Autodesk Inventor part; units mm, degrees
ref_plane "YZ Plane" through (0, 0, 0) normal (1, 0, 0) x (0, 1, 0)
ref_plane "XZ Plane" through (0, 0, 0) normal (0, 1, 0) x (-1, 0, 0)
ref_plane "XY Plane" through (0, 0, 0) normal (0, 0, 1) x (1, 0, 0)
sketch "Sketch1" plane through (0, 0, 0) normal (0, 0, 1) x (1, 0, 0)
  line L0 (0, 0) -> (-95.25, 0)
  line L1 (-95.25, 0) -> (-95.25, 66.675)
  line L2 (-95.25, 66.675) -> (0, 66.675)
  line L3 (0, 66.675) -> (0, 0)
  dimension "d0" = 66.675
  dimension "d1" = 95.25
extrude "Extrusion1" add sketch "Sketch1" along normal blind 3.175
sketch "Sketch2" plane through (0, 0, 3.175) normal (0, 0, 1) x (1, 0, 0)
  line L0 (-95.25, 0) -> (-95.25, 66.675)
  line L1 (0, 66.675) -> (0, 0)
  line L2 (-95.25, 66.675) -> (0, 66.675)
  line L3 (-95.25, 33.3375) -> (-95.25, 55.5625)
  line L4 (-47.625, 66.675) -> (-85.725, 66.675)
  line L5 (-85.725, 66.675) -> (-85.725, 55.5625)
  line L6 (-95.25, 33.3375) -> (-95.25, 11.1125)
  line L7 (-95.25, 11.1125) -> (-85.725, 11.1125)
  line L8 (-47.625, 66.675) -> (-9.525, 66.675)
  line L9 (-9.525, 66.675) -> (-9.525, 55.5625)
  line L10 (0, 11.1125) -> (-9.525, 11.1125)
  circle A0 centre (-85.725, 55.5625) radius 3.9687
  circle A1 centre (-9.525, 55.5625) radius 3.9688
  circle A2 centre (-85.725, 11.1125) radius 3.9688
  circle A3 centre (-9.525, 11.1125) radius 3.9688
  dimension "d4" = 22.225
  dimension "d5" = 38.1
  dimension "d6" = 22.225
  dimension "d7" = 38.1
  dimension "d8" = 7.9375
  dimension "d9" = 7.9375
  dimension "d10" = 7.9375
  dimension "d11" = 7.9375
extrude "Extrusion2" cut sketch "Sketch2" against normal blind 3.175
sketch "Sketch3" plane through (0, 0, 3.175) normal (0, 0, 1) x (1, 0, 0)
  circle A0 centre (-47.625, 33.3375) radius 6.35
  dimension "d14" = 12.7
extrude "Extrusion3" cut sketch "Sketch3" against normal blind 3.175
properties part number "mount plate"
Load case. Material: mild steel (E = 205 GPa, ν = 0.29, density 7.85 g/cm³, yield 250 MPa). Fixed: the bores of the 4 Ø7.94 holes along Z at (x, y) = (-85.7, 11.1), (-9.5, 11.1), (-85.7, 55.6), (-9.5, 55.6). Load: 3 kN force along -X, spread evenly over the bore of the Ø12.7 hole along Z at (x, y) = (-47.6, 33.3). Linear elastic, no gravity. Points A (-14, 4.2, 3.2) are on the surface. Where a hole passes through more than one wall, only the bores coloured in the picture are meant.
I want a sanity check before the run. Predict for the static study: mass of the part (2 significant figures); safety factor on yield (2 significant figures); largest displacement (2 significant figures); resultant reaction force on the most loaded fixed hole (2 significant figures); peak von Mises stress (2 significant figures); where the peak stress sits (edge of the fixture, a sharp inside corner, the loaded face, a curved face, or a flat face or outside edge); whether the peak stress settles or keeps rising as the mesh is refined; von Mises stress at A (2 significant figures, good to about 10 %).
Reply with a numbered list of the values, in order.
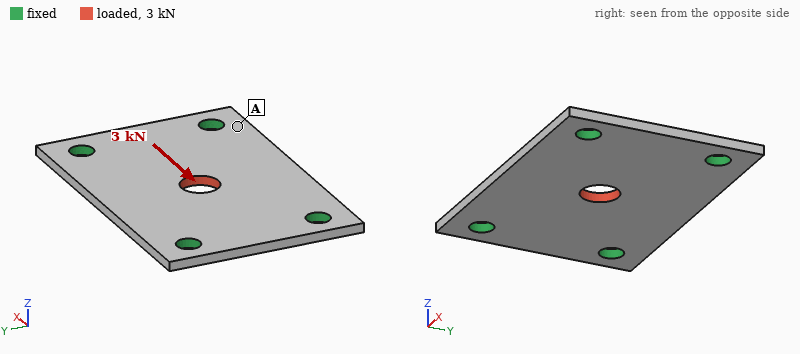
1. 150 g
2. 6.1
3. 2.7 µm
4. 790 N
5. 41 MPa
6. the loaded face
7. settles
8. 5.0 MPa
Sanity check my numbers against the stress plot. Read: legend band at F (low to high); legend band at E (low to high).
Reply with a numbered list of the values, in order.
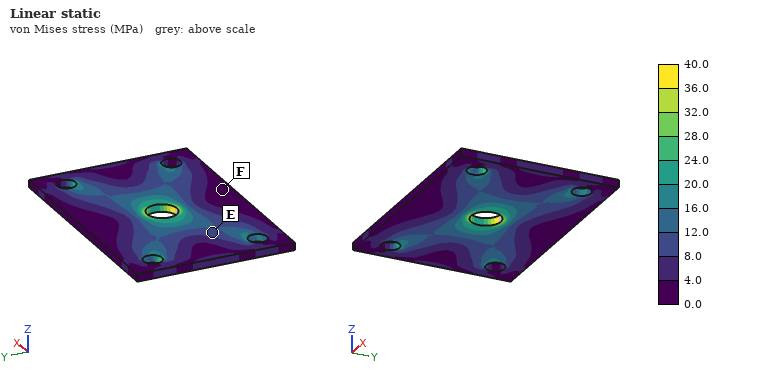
1. 0.0 to 4.0 MPa
2. 8.0 to 12.0 MPa
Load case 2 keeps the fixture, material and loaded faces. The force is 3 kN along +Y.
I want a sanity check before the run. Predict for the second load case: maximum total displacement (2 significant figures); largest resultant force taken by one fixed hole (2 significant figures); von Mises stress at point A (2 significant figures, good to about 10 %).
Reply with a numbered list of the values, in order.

1. 4.7 µm
2. 920 N
3. 8.8 MPa
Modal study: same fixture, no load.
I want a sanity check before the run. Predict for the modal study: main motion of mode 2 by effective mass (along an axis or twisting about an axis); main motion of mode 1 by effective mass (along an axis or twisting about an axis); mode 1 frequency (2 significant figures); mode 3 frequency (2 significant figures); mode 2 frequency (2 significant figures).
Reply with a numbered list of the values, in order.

1. twisting about X
2. along Z
3. 3000 Hz
4. 6000 Hz
5. 3900 Hz
